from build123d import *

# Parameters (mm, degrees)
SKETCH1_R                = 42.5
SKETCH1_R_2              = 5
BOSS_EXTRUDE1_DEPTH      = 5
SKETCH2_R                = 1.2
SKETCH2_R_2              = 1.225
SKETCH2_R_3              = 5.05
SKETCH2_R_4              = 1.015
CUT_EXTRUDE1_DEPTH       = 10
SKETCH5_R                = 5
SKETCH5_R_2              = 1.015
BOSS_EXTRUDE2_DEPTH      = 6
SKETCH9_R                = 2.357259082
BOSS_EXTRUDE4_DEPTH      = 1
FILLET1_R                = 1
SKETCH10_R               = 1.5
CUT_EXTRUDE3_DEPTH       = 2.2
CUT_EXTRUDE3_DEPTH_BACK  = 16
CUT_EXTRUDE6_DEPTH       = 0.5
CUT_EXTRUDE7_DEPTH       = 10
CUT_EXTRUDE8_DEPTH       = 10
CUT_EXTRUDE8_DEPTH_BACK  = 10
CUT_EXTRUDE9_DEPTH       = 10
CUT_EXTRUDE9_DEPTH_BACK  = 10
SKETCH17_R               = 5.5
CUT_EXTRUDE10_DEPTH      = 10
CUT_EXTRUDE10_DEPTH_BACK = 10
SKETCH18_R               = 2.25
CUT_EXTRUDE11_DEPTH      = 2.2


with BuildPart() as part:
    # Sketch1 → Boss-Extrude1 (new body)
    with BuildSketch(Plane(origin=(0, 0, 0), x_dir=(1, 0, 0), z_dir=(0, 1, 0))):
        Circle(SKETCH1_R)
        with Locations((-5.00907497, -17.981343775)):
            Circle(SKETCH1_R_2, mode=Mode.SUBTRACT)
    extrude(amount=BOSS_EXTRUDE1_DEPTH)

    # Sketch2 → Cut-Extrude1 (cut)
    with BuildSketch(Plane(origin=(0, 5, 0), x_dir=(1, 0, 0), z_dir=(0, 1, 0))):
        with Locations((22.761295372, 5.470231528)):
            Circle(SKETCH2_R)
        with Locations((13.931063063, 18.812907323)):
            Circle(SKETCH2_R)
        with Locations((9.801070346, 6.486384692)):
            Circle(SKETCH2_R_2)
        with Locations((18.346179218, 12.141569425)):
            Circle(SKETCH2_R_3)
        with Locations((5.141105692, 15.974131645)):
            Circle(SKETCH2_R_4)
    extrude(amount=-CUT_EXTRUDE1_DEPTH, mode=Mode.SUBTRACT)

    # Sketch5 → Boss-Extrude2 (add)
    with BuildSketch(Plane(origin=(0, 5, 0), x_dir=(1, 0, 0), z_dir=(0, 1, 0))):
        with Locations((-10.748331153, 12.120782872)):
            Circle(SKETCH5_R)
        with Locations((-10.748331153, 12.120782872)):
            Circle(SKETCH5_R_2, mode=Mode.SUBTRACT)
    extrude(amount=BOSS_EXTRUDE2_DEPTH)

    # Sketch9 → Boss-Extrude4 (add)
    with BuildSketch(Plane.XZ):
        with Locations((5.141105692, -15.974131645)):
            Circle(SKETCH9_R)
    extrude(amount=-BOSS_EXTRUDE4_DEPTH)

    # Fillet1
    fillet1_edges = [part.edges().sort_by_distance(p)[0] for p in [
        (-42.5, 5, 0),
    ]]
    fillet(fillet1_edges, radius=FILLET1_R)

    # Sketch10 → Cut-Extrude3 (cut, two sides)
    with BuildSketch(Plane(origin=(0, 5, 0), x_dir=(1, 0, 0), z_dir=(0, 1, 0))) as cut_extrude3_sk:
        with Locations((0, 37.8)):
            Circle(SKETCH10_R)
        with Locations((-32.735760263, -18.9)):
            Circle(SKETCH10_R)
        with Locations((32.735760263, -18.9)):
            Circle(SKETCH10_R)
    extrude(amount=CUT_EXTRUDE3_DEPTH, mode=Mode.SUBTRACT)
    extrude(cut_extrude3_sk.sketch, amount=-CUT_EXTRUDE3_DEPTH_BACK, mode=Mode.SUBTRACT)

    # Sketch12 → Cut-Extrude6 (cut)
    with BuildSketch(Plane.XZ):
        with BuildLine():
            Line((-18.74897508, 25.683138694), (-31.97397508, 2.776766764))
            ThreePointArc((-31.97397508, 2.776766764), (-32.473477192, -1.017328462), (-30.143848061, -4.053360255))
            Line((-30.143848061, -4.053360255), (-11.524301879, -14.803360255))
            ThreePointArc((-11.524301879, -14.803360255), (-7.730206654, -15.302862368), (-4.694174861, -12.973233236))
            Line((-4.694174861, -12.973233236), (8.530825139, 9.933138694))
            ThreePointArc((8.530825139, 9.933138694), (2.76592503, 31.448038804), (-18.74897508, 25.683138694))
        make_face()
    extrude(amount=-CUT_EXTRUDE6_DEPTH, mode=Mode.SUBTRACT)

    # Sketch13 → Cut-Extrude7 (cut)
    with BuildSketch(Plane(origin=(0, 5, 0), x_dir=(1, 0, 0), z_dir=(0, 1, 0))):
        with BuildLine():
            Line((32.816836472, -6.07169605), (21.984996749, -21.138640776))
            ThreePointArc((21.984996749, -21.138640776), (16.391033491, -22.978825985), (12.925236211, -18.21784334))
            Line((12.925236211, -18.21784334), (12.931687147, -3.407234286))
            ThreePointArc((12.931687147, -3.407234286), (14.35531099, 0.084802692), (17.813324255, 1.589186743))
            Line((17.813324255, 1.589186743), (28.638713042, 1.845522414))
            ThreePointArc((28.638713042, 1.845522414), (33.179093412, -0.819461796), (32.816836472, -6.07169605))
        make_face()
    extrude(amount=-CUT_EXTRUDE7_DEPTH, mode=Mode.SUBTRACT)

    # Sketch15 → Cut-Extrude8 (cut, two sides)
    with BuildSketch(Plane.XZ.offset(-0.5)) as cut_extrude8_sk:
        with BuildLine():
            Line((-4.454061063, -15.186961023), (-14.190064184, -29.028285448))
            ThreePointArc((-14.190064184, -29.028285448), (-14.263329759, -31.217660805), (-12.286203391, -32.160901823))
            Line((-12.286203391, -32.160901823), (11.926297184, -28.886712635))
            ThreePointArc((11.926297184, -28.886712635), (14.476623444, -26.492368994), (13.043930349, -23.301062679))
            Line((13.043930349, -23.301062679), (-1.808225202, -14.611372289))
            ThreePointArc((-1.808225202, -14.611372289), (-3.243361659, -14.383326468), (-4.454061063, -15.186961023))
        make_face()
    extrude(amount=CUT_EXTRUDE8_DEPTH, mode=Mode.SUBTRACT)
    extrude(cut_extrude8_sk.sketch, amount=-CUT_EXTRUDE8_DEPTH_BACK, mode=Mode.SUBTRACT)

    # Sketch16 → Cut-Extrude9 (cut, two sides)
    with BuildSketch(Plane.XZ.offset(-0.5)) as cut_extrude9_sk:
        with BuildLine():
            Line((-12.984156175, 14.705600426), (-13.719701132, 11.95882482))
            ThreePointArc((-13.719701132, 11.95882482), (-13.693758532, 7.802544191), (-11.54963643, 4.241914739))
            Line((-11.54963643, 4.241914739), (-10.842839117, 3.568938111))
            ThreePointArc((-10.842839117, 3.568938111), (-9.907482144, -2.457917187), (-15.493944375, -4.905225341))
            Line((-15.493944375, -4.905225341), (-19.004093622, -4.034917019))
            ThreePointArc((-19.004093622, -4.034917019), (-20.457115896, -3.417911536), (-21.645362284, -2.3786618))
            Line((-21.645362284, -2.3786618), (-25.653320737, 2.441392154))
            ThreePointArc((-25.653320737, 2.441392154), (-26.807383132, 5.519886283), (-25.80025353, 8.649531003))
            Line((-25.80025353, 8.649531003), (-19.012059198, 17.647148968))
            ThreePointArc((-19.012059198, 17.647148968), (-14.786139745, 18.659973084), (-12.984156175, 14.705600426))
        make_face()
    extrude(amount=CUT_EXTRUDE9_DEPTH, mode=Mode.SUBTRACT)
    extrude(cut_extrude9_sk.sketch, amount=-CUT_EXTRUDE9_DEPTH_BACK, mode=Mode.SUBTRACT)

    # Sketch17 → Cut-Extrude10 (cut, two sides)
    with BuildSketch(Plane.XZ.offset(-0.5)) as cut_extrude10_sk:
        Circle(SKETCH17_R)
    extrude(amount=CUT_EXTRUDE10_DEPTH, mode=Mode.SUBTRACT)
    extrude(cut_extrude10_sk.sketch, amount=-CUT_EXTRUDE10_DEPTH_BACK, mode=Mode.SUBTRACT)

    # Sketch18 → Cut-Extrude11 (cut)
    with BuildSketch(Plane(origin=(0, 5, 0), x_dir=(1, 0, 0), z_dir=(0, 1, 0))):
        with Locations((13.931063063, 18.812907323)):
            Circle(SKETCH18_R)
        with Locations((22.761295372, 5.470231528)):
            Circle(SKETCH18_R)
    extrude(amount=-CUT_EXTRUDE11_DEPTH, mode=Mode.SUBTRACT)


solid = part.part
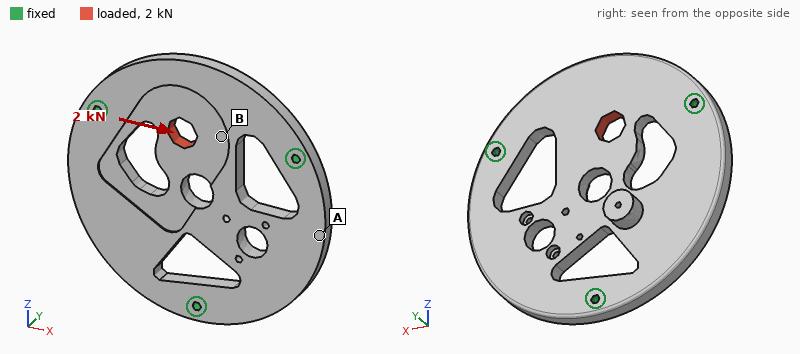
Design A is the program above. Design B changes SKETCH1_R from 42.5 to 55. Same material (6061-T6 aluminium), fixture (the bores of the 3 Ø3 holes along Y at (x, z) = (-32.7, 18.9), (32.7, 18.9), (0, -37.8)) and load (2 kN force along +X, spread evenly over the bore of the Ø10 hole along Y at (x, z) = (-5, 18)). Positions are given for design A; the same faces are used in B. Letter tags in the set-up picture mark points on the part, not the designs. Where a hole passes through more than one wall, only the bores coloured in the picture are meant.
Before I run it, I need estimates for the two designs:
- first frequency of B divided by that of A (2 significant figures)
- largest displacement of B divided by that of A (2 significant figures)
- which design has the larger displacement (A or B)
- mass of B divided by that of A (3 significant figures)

0.66
0.88
A
1.87
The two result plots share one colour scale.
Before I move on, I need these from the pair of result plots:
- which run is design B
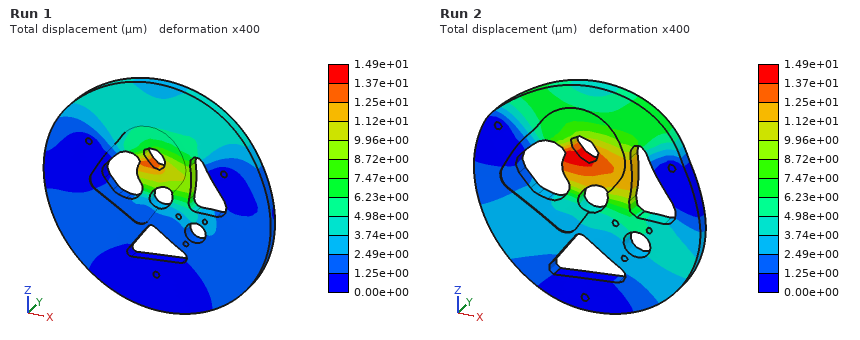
Run 1
